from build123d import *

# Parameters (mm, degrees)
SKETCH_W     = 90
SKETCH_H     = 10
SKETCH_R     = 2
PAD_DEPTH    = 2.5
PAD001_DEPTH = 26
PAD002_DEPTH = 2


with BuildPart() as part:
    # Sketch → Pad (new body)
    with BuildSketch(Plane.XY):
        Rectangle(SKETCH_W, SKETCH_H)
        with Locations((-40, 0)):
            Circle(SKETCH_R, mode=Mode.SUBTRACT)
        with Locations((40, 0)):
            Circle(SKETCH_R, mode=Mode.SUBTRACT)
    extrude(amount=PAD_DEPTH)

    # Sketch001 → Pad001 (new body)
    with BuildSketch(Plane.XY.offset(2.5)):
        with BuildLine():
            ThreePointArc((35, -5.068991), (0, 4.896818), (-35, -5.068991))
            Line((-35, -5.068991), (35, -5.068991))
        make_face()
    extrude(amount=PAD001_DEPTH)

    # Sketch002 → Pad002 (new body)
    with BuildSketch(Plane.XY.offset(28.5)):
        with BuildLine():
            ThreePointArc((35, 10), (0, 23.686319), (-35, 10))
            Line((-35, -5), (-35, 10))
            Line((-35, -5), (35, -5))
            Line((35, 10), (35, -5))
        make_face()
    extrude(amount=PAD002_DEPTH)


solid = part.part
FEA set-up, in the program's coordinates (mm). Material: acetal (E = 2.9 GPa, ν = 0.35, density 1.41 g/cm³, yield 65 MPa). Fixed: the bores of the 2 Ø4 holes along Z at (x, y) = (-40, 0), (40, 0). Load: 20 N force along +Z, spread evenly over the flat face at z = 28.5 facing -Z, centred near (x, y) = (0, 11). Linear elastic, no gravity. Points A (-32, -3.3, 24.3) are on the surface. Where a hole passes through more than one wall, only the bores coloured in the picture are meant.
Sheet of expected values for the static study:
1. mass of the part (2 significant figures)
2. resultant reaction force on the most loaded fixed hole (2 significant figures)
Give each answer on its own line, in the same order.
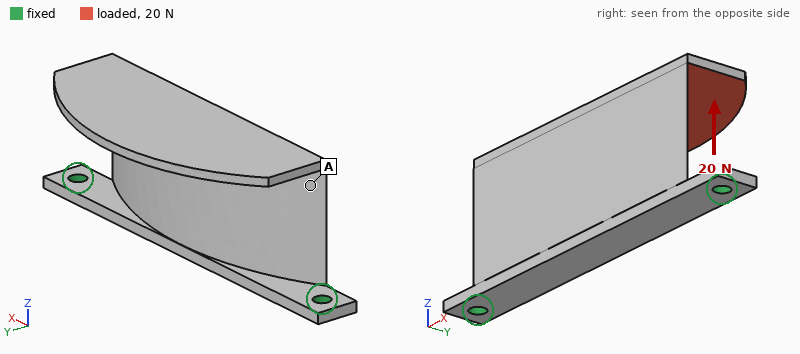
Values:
25 g
12 N
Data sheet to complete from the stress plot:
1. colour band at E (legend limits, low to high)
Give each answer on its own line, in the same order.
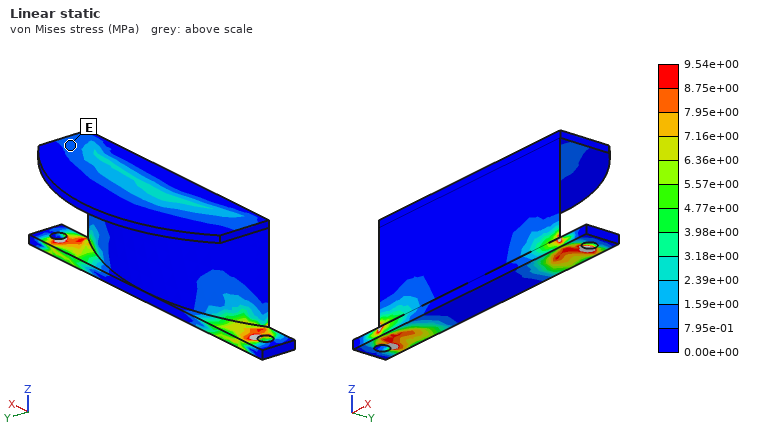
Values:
7.95e-01 to 1.59e+00 MPa
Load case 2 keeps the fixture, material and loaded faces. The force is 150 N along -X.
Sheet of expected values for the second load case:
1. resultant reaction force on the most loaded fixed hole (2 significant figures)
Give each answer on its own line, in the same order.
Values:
99 N
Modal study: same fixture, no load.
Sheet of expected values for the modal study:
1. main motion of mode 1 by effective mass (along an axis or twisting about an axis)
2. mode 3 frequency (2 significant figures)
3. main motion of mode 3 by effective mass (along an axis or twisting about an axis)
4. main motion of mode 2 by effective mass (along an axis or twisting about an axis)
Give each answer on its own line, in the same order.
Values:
along Y
1100 Hz
along X
along Z
